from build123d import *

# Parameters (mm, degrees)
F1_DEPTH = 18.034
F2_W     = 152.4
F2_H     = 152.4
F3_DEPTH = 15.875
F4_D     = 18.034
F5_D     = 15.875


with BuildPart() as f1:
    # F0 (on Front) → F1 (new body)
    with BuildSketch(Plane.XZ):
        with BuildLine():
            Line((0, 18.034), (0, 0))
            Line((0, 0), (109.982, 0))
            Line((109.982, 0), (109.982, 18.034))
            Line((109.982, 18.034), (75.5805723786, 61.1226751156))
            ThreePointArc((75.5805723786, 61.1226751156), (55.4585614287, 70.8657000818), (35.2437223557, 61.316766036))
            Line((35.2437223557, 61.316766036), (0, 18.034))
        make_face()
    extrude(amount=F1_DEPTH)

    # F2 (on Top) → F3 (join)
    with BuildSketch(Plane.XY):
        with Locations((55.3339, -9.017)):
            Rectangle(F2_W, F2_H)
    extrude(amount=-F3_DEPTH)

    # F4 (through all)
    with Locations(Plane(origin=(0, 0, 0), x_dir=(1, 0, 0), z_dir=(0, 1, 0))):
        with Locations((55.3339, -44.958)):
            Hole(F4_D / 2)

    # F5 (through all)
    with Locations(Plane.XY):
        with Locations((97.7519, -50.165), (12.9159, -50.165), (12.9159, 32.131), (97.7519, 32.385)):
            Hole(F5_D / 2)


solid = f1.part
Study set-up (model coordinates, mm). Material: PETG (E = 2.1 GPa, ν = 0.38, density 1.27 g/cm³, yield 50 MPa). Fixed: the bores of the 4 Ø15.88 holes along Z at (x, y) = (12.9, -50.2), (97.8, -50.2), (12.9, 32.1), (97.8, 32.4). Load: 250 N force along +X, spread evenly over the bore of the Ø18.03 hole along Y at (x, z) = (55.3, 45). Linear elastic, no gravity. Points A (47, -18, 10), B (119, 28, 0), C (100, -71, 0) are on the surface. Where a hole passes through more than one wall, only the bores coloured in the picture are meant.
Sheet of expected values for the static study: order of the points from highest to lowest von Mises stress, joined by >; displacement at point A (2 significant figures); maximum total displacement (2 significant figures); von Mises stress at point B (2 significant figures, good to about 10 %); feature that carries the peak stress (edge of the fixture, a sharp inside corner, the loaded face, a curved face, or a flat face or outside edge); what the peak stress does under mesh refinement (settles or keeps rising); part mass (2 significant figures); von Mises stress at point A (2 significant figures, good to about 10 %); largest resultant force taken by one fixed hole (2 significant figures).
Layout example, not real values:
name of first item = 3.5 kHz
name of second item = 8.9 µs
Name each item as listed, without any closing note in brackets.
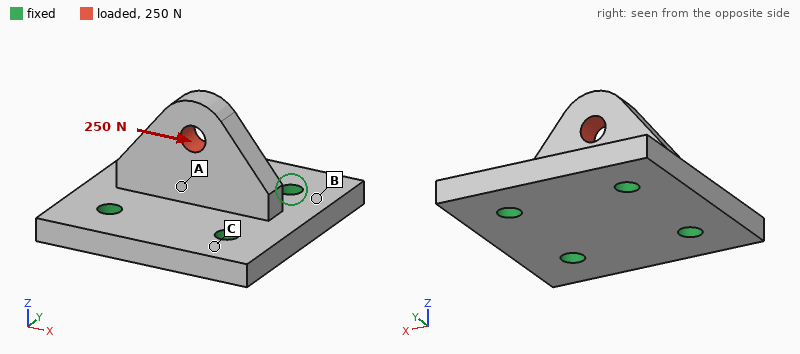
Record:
order of the points from highest to lowest von Mises stress, joined by > = A > B > C
displacement at point A = 9.1 µm
maximum total displacement = 34 µm
von Mises stress at point B = 0.16 MPa
feature that carries the peak stress = edge of the fixture
what the peak stress does under mesh refinement = keeps rising
part mass = 570 g
von Mises stress at point A = 0.24 MPa
largest resultant force taken by one fixed hole = 97 N
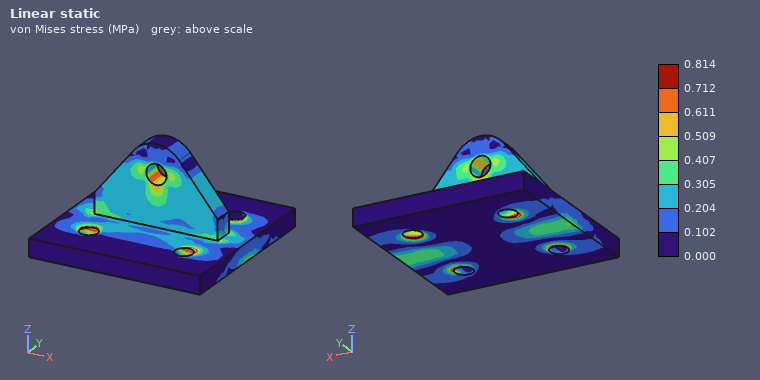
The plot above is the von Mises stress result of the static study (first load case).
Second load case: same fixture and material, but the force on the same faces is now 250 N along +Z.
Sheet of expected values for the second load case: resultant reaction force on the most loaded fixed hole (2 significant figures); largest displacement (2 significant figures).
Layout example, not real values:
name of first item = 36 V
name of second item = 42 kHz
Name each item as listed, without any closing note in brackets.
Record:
resultant reaction force on the most loaded fixed hole = 64 N
largest displacement = 17 µm
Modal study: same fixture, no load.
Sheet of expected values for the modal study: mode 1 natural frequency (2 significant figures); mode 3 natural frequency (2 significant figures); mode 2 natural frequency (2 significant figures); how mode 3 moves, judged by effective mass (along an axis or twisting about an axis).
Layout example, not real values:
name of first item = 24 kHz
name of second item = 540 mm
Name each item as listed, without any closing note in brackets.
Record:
mode 1 natural frequency = 860 Hz
mode 3 natural frequency = 1700 Hz
mode 2 natural frequency = 1600 Hz
how mode 3 moves, judged by effective mass = along Z
